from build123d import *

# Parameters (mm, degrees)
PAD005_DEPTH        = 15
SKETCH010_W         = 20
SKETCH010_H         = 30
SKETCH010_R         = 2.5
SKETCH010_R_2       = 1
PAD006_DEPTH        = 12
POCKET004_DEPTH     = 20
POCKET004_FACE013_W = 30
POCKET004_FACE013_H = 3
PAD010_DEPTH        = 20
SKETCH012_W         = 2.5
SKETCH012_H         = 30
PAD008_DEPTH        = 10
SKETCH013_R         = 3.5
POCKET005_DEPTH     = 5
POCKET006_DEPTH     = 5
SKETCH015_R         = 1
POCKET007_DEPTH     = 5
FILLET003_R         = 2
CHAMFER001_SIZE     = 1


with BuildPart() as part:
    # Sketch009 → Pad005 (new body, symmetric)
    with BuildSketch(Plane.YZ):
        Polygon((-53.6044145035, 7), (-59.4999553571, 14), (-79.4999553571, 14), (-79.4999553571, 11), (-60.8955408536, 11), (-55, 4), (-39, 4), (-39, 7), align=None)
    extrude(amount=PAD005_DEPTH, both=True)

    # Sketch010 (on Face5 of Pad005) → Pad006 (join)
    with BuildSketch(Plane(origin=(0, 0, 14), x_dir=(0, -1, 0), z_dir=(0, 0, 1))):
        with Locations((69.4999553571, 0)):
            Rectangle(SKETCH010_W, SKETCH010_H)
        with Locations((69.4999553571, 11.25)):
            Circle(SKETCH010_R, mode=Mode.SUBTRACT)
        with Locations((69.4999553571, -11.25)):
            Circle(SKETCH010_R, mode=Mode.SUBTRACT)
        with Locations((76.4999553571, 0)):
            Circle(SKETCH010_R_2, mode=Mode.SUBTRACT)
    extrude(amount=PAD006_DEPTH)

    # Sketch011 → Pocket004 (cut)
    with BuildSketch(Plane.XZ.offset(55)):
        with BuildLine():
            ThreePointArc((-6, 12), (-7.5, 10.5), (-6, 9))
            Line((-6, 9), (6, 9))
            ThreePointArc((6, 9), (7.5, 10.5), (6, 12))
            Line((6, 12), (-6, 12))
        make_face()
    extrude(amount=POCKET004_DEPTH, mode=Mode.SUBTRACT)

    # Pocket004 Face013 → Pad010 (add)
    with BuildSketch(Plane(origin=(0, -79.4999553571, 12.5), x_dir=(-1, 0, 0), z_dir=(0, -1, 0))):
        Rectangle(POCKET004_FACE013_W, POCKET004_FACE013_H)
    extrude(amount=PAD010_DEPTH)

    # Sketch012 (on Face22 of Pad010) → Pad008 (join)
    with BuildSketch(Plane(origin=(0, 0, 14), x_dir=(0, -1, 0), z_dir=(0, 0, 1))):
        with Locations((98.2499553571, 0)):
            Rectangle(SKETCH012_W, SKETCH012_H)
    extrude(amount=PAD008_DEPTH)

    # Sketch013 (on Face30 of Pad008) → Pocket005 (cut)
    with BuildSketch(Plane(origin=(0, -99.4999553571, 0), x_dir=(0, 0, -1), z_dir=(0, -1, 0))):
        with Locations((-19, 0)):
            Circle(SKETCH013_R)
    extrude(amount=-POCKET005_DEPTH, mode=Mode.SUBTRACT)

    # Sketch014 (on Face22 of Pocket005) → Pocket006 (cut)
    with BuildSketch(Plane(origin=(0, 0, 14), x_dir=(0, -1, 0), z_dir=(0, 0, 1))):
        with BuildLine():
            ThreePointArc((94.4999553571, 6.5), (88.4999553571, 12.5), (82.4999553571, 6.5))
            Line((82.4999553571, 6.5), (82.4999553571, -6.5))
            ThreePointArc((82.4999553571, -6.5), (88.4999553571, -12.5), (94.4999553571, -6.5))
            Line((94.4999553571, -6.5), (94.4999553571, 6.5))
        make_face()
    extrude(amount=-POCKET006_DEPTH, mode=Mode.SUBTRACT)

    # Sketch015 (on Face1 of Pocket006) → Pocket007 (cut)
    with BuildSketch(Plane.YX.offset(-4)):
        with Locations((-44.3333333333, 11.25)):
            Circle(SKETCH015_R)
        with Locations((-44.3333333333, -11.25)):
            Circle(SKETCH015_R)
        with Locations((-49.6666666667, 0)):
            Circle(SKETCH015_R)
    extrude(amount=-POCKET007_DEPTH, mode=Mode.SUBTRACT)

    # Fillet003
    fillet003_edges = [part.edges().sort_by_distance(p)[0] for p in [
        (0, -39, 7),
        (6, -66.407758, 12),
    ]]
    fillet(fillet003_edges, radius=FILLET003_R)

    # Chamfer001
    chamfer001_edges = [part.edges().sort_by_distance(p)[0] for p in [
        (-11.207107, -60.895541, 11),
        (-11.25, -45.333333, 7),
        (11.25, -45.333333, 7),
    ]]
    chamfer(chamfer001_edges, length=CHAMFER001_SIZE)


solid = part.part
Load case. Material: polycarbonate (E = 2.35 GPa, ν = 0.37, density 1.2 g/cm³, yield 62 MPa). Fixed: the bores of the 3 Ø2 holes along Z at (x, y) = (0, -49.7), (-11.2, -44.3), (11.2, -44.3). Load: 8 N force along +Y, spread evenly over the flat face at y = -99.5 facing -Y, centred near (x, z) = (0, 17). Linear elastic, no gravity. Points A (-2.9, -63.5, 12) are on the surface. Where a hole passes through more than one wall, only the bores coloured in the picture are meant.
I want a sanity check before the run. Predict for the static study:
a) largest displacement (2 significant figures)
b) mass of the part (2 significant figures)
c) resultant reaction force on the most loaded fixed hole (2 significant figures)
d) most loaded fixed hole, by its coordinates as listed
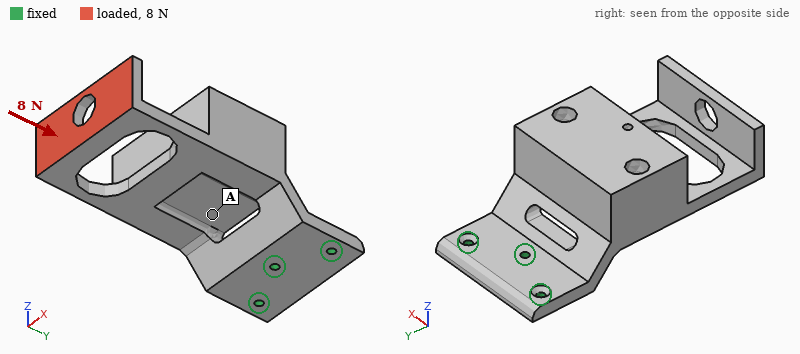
0.77 mm
14 g
7.7 N
(0, -49.7)
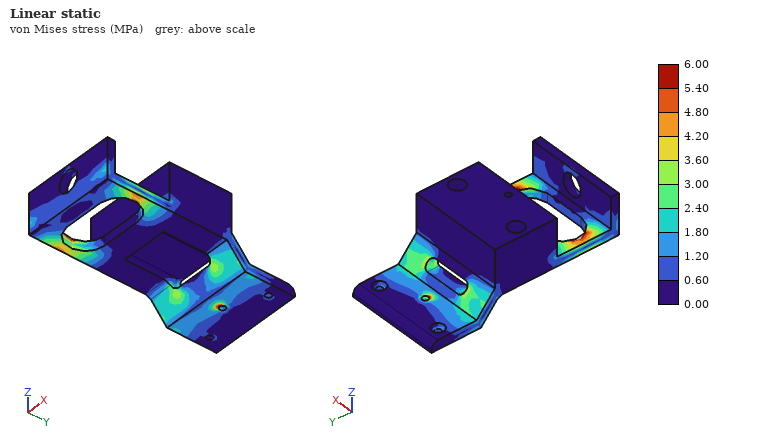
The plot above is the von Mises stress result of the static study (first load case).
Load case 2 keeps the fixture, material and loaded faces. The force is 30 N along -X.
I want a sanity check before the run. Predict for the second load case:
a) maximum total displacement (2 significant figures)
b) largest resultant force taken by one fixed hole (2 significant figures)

0.61 mm
65 N
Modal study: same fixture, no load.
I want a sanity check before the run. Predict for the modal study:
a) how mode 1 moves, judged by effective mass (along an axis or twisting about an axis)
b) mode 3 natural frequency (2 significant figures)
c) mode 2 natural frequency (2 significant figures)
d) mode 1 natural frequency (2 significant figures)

along Z
680 Hz
660 Hz
160 Hz
